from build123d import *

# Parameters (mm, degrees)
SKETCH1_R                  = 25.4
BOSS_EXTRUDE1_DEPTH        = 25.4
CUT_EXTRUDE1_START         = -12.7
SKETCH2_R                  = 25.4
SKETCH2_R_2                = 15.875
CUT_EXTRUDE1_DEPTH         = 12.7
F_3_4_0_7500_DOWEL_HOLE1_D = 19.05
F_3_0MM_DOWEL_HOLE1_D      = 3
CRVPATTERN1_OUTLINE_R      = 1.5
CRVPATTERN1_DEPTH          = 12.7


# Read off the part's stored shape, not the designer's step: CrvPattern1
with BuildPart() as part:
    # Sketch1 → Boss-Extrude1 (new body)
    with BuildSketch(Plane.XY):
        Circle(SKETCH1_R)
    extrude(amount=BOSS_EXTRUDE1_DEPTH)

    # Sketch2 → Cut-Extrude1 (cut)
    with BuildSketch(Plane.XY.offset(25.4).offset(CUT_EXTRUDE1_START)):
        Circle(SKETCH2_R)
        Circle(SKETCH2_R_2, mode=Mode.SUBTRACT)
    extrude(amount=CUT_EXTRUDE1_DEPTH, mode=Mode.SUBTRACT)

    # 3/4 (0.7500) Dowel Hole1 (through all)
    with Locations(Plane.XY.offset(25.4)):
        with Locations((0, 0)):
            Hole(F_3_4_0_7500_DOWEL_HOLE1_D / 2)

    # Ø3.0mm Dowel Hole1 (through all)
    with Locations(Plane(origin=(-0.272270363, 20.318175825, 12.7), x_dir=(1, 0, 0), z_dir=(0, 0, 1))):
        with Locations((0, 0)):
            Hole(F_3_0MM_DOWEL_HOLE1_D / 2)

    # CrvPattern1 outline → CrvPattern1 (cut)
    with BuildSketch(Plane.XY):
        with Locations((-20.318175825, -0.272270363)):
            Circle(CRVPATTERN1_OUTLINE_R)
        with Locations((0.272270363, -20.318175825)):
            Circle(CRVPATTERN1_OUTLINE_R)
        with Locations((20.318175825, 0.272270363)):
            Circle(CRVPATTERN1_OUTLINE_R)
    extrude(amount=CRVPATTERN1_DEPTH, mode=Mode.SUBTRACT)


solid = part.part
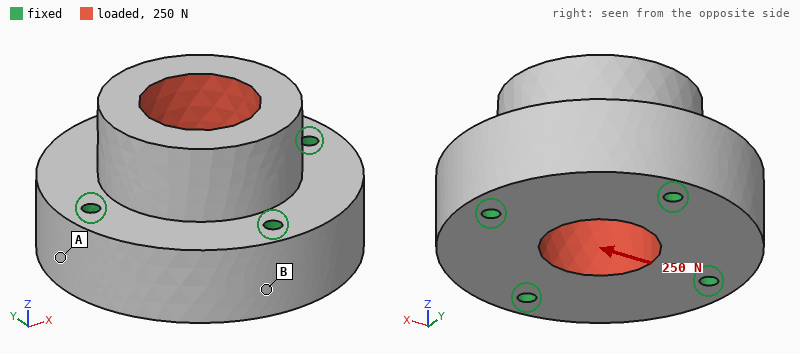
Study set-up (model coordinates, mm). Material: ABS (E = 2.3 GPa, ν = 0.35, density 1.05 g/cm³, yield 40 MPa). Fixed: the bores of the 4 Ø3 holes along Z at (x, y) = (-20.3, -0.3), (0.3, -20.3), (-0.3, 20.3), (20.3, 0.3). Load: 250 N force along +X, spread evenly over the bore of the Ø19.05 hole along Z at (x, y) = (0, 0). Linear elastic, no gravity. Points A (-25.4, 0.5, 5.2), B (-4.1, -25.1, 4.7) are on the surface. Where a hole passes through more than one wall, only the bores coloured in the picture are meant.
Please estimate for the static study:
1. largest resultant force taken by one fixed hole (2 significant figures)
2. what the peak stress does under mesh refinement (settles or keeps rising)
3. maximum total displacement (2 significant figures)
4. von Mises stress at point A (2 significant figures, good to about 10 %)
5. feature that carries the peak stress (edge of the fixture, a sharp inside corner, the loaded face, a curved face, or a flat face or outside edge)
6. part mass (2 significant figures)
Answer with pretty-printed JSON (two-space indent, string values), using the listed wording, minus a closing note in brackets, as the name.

{
  "largest resultant force taken by one fixed hole": "79 N",
  "what the peak stress does under mesh refinement": "keeps rising",
  "maximum total displacement": "9.3 µm",
  "von Mises stress at point A": "0.28 MPa",
  "feature that carries the peak stress": "edge of the fixture",
  "part mass": "30 g"
}
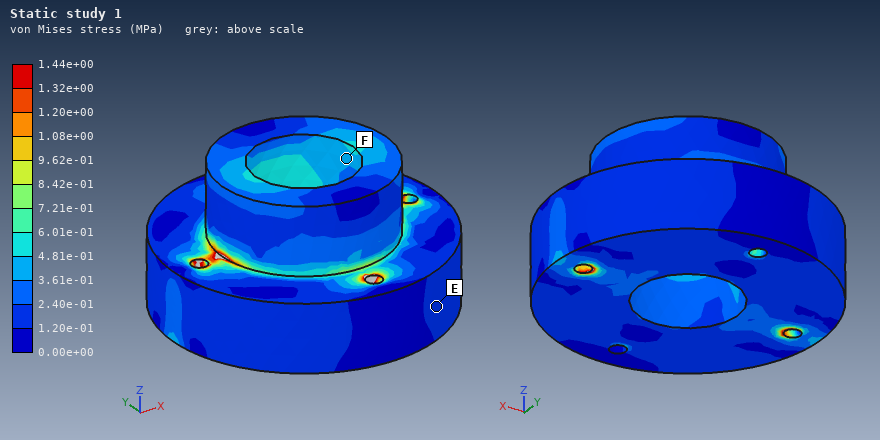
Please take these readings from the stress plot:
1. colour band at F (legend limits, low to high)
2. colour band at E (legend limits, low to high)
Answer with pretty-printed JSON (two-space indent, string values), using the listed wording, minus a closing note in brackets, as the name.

{
  "colour band at F": "3.61e-01 to 4.81e-01 MPa",
  "colour band at E": "1.20e-01 to 2.40e-01 MPa"
}
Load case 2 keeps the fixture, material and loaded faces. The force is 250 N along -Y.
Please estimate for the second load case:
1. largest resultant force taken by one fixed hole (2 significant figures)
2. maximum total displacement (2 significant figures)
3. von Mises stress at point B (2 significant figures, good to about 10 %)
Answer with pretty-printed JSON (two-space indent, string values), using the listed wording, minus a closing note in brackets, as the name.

{
  "largest resultant force taken by one fixed hole": "79 N",
  "maximum total displacement": "9.3 µm",
  "von Mises stress at point B": "0.17 MPa"
}
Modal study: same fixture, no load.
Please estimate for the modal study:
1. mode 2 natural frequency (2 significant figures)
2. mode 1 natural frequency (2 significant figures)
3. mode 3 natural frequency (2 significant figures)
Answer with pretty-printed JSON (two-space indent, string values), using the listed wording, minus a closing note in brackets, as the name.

{
  "mode 2 natural frequency": "7900 Hz",
  "mode 1 natural frequency": "7900 Hz",
  "mode 3 natural frequency": "8500 Hz"
}
